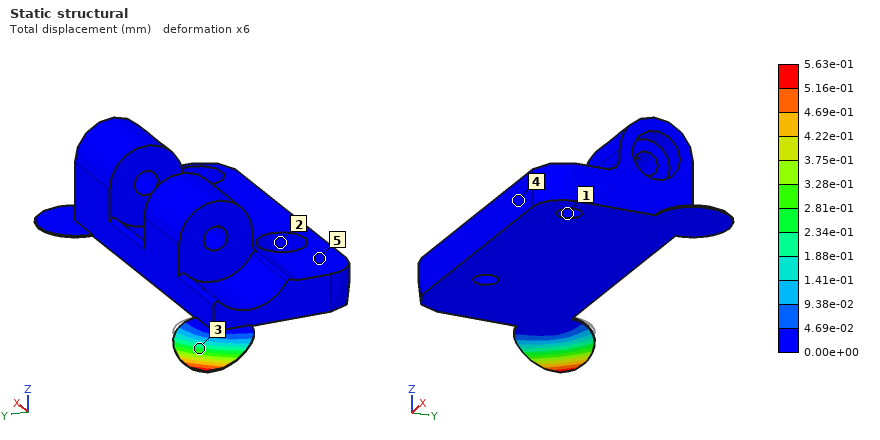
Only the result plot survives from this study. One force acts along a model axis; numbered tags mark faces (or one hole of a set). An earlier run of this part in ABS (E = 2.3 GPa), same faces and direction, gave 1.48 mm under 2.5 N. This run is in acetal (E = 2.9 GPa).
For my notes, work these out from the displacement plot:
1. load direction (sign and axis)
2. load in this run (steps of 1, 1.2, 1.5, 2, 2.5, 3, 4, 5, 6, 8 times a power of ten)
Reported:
-Z
1.2 N
